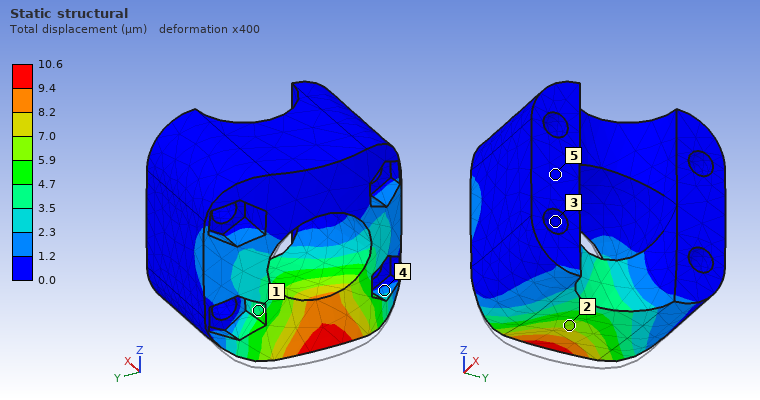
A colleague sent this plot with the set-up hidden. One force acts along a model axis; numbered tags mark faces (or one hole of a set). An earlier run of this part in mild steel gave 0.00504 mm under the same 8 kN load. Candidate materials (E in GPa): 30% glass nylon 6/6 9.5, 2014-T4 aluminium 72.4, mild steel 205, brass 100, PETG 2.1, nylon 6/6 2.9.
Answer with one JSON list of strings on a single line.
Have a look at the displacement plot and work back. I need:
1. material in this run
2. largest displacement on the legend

["brass", "10.6 µm"]
